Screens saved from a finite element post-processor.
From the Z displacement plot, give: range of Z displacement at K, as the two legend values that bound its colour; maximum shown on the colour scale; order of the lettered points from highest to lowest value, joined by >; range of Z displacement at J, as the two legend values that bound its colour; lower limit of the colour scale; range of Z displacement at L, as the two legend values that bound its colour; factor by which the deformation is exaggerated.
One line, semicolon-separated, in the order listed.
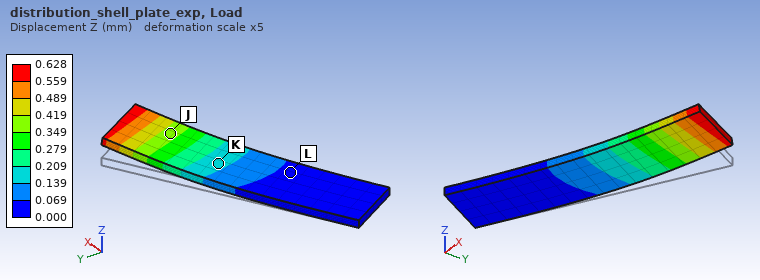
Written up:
0.139 to 0.209 mm; 0.628 mm; J > K > L; 0.349 to 0.419 mm; 0.000 mm; 0.000 to 0.069 mm; 5
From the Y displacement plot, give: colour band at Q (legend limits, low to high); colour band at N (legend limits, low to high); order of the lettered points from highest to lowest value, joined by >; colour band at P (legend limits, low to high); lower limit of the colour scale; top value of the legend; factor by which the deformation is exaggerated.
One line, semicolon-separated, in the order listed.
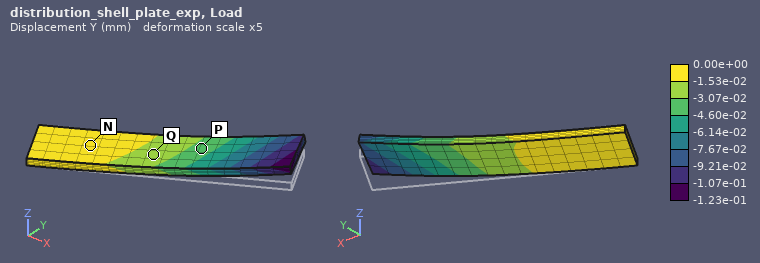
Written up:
-3.07e-02 to -1.53e-02 mm; -1.53e-02 to 0.00e+00 mm; N > Q > P; -4.60e-02 to -3.07e-02 mm; -1.23e-01 mm; 0.00e+00 mm; 5
